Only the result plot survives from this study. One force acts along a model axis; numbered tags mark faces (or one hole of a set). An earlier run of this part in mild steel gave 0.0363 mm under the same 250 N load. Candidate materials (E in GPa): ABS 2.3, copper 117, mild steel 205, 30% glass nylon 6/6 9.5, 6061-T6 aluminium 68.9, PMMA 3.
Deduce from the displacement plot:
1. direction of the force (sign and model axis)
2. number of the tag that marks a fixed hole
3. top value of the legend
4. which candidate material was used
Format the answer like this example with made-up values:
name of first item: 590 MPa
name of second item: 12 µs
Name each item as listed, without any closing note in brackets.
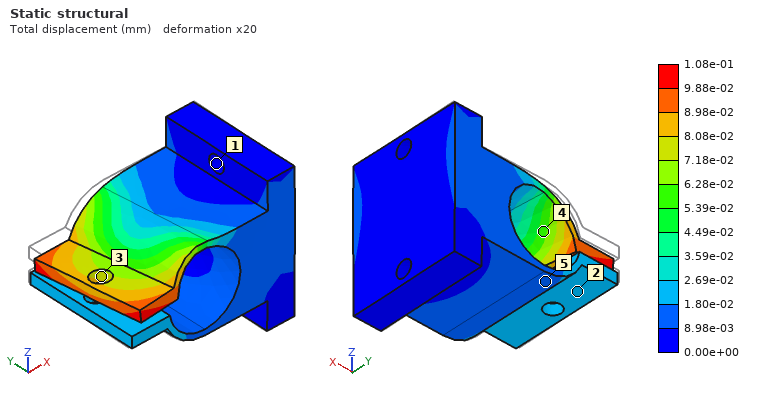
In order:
direction of the force: -Y
number of the tag that marks a fixed hole: 1
top value of the legend: 1.08e-01 mm
which candidate material was used: 6061-T6 aluminium
